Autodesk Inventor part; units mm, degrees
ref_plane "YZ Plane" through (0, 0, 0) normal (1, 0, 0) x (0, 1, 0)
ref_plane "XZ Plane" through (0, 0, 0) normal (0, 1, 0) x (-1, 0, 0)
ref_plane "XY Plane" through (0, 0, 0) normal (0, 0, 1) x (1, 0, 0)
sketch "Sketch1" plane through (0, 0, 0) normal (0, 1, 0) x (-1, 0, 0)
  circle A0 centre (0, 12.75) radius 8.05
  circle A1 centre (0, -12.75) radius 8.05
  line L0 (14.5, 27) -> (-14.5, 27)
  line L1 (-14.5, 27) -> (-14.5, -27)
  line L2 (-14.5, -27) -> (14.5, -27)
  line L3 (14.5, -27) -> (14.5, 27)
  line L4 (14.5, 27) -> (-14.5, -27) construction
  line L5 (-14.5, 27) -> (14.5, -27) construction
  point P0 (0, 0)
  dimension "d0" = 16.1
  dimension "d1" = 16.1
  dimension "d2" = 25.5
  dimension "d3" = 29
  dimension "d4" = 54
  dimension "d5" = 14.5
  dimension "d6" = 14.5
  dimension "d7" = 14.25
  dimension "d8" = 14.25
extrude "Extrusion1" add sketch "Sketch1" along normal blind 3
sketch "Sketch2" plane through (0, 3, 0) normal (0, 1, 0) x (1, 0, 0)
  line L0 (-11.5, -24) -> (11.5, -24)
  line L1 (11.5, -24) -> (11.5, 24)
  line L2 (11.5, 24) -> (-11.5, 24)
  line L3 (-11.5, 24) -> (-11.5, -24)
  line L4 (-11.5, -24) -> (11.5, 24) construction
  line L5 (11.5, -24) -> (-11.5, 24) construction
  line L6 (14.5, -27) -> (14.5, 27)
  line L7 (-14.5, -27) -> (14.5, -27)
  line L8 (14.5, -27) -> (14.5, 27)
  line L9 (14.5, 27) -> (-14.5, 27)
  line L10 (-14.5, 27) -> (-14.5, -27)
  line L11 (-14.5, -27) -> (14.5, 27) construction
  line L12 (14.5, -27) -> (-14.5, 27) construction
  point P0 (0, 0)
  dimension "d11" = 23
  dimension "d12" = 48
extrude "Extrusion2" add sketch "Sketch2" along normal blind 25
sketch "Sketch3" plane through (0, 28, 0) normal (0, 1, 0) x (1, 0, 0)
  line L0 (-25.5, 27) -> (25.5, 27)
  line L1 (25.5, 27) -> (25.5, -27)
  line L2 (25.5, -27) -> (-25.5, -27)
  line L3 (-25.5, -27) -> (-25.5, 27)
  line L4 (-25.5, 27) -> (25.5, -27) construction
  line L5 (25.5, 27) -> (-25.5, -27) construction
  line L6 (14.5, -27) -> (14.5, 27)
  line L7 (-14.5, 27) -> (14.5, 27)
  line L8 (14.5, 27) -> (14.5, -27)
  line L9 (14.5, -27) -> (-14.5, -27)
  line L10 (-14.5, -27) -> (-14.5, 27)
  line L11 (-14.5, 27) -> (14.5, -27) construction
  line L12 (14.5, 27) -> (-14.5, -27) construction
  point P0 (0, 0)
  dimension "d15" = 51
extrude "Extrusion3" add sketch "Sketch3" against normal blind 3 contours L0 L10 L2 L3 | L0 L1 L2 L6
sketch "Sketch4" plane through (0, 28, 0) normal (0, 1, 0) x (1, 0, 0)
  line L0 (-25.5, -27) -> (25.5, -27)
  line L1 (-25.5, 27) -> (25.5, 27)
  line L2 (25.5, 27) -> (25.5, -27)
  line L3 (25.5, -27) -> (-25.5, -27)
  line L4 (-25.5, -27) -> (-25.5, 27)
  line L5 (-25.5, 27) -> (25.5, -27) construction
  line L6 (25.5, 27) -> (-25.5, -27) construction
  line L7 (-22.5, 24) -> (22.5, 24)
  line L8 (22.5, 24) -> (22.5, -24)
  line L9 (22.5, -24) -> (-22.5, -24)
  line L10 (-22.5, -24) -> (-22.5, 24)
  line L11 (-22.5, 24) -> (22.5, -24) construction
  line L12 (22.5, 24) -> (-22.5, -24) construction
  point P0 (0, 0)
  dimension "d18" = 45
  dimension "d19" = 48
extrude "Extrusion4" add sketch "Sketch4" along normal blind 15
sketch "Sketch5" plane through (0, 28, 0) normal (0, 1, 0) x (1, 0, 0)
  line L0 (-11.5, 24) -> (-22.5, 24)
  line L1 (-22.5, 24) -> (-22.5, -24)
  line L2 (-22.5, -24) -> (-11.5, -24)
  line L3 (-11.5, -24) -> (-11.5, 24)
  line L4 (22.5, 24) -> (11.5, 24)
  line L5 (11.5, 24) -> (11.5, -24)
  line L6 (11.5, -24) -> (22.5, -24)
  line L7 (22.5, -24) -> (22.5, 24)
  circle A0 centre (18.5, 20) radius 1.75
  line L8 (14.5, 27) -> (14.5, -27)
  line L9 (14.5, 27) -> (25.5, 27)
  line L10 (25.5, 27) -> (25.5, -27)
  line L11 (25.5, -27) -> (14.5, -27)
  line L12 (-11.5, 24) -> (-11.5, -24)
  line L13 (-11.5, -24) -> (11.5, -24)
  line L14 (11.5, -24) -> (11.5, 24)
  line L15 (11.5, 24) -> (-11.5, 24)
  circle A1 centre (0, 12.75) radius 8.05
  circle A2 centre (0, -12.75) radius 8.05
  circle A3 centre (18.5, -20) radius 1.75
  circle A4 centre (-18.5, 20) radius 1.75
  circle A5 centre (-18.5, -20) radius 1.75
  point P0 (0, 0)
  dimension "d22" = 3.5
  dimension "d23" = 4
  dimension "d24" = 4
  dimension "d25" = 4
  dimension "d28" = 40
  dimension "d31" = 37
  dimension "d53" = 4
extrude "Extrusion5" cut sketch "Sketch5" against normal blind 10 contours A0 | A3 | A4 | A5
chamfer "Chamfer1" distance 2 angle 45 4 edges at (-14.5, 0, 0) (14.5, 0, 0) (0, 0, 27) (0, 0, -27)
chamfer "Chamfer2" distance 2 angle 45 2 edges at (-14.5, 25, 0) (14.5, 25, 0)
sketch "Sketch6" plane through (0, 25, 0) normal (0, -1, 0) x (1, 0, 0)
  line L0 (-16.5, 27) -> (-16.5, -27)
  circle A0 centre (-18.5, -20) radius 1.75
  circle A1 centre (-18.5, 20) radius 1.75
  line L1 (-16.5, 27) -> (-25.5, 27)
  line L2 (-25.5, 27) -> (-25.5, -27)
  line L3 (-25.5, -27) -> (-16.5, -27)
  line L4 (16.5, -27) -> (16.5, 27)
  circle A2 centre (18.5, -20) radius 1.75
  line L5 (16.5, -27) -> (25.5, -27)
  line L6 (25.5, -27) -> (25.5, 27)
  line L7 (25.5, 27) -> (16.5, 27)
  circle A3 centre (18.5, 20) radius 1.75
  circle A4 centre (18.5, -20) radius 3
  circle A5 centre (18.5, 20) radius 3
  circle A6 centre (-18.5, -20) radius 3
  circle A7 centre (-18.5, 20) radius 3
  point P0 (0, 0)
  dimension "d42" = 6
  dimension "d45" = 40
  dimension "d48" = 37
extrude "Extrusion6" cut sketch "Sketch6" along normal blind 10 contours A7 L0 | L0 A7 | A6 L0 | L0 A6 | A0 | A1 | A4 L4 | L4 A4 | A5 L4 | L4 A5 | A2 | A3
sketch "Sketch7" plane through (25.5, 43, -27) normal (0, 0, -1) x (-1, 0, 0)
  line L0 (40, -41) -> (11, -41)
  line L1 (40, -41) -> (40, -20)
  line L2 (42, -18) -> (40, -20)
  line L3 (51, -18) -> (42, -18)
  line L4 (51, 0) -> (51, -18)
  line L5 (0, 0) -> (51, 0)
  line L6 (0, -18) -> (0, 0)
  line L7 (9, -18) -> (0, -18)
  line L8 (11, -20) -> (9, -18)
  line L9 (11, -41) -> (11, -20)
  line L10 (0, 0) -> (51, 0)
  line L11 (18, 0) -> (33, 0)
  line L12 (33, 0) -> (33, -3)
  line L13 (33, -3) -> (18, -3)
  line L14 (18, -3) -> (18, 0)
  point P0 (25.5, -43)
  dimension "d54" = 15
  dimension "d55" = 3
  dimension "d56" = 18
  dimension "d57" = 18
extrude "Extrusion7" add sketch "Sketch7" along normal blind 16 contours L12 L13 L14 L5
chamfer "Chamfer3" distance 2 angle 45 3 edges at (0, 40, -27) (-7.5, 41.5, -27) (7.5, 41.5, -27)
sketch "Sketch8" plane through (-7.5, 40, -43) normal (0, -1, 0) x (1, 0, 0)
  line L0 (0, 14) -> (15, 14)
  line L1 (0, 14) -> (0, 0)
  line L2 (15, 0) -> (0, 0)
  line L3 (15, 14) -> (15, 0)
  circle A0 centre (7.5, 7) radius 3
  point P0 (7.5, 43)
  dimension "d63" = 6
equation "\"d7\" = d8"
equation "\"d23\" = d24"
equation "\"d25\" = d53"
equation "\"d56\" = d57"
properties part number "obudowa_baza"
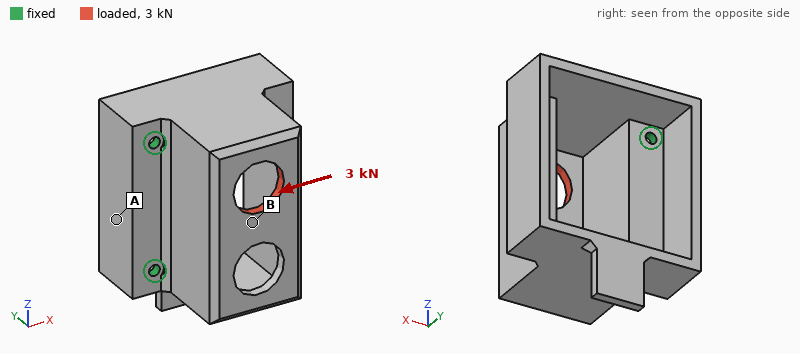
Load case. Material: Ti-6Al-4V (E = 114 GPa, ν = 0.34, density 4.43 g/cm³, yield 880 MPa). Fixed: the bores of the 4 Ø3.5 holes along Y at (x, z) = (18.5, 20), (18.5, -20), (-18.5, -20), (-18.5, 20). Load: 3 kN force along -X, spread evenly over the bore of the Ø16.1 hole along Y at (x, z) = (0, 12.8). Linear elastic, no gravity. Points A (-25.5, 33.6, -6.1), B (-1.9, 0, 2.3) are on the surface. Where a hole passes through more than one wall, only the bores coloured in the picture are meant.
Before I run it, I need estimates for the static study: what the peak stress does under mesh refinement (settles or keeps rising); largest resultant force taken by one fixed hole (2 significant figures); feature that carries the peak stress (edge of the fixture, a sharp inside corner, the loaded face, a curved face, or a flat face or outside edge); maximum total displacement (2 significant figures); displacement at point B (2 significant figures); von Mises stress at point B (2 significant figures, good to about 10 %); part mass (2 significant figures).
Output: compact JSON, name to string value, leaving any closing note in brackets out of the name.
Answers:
{"what the peak stress does under mesh refinement": "keeps rising", "largest resultant force taken by one fixed hole": "1.7 kN", "feature that carries the peak stress": "edge of the fixture", "maximum total displacement": "45 µm", "displacement at point B": "40 µm", "von Mises stress at point B": "35 MPa", "part mass": "120 g"}
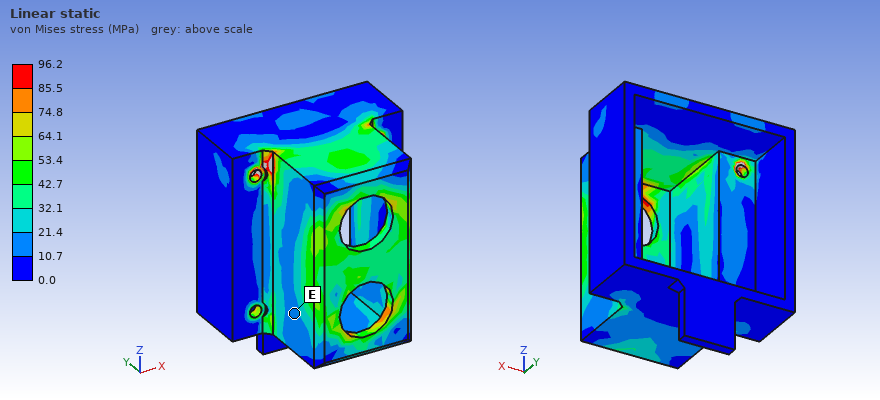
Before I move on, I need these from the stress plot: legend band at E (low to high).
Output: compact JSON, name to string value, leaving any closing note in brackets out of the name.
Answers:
{"legend band at E": "10.7 to 21.4 MPa"}
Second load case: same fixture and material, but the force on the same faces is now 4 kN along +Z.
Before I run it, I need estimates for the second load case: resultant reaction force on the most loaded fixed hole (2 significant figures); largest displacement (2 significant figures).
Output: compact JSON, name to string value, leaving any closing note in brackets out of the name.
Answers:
{"resultant reaction force on the most loaded fixed hole": "1.6 kN", "largest displacement": "31 µm"}
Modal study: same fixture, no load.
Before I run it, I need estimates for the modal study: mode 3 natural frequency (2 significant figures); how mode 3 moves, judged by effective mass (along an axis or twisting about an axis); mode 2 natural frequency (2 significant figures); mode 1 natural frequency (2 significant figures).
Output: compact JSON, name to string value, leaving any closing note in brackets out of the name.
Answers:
{"mode 3 natural frequency": "9000 Hz", "how mode 3 moves, judged by effective mass": "along X", "mode 2 natural frequency": "8500 Hz", "mode 1 natural frequency": "5200 Hz"}
